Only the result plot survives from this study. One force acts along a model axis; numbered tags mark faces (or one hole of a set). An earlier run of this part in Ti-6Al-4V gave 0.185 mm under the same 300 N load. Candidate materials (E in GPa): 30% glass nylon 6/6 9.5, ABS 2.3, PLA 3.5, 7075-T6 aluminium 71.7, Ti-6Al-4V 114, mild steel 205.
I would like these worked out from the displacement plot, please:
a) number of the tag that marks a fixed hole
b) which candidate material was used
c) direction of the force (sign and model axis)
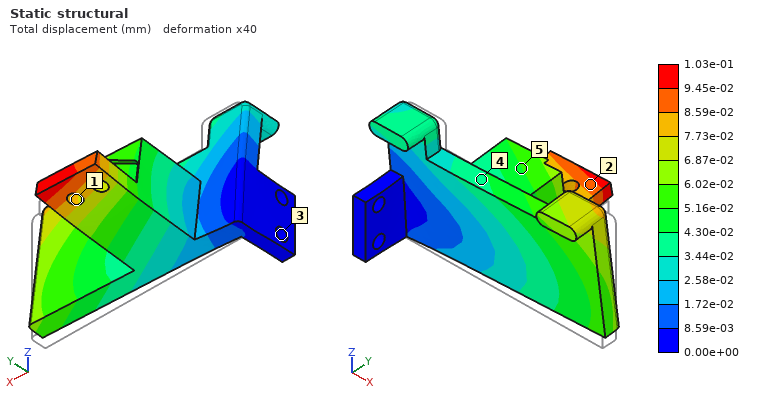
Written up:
3
mild steel
+Z
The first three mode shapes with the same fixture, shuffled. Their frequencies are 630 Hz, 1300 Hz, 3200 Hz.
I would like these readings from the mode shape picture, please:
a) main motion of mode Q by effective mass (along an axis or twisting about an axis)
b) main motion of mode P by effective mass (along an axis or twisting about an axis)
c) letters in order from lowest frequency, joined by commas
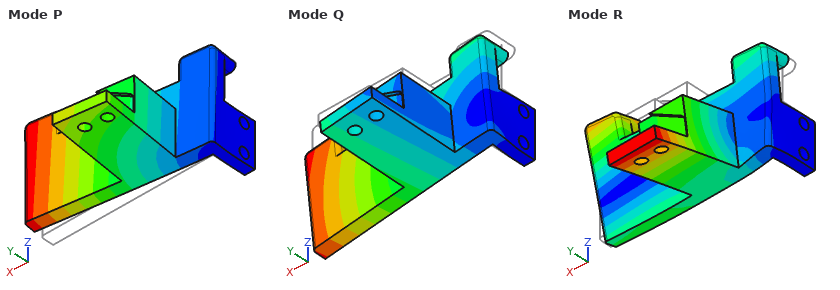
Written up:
along Z
along Y
P, Q, R
